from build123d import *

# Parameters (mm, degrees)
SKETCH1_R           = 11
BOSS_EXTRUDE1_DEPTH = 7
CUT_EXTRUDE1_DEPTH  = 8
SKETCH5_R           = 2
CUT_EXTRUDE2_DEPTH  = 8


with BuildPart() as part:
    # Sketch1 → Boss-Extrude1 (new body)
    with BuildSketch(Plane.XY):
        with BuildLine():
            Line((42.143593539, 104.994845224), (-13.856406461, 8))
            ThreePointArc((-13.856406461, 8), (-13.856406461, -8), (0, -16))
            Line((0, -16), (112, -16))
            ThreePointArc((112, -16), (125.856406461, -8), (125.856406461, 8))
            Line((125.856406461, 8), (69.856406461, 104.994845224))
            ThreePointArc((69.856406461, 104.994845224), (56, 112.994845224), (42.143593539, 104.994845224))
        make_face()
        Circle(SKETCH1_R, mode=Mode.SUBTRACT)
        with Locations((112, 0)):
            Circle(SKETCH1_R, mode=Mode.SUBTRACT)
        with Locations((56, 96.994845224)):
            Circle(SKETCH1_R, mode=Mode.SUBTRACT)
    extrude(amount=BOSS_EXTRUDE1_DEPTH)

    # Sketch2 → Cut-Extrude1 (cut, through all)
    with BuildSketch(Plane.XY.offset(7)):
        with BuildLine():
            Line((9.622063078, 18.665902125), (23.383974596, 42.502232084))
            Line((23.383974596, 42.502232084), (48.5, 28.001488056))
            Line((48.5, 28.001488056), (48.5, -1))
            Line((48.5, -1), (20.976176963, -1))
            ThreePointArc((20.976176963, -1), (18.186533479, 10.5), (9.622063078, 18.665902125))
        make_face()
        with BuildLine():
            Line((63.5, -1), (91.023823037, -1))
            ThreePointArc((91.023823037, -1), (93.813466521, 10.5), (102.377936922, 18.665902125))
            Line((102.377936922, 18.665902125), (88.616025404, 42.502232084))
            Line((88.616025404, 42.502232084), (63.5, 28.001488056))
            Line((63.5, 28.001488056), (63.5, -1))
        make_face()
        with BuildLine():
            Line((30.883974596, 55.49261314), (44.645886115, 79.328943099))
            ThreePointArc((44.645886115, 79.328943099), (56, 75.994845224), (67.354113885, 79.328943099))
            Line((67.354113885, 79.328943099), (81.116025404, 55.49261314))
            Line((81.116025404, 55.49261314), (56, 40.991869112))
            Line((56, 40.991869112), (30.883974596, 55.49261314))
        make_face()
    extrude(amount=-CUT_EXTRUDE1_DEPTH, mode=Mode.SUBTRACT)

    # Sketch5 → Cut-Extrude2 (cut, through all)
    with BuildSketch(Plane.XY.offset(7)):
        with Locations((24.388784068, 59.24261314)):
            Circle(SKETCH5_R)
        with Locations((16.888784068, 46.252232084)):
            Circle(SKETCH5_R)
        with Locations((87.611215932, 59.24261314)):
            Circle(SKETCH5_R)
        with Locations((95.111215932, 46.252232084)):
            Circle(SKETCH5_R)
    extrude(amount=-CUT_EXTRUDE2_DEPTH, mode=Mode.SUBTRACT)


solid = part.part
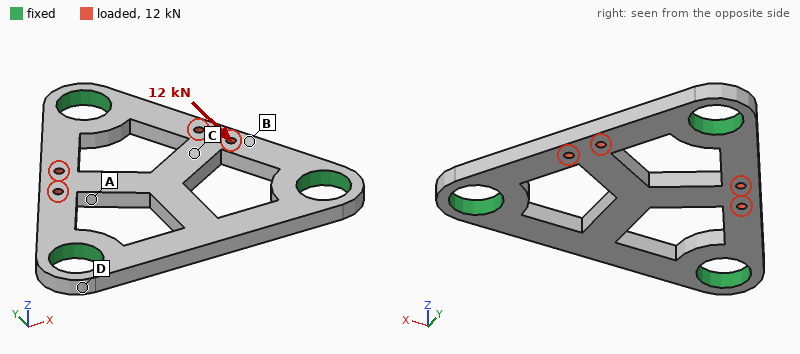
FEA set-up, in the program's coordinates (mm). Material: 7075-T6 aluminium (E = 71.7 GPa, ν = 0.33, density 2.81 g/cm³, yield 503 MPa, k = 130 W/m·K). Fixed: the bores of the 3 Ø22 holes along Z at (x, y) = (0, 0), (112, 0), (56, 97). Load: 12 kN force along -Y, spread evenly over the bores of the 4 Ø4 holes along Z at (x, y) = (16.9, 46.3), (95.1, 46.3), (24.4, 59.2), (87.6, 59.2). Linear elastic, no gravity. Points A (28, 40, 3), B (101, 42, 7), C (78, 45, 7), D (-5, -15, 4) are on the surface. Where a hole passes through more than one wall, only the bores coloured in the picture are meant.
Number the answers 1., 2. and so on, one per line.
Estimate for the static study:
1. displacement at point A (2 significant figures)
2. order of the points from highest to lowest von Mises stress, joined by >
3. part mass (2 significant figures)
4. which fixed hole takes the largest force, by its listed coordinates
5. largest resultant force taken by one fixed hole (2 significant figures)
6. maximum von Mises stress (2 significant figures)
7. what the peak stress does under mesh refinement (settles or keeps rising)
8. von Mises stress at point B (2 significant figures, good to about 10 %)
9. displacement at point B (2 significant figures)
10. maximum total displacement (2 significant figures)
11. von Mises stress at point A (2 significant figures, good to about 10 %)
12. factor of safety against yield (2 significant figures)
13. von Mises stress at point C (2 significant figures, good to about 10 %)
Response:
1. 29 µm
2. B > A > C > D
3. 140 g
4. (56, 97)
5. 4.9 kN
6. 78 MPa
7. settles
8. 34 MPa
9. 21 µm
10. 38 µm
11. 26 MPa
12. 6.4
13. 19 MPa
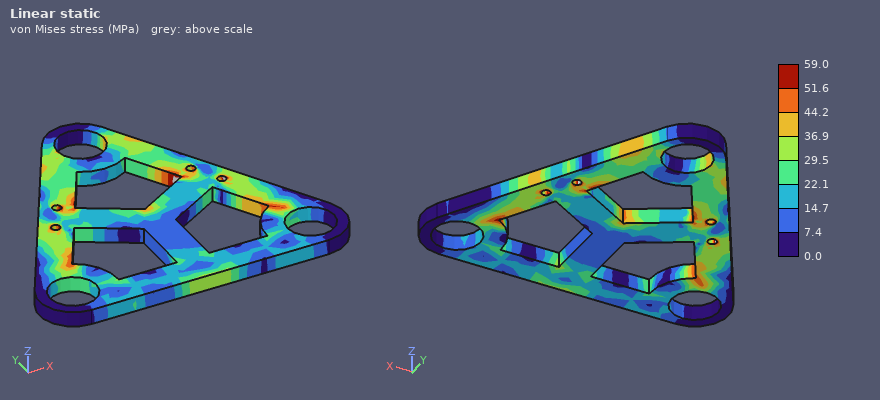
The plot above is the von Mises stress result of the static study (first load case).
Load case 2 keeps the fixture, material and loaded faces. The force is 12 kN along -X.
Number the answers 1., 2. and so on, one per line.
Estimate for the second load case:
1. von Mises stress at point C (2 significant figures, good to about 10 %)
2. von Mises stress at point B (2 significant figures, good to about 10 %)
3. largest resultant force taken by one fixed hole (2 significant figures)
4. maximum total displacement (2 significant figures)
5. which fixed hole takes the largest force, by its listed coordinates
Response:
1. 27 MPa
2. 48 MPa
3. 5.4 kN
4. 99 µm
5. (56, 97)
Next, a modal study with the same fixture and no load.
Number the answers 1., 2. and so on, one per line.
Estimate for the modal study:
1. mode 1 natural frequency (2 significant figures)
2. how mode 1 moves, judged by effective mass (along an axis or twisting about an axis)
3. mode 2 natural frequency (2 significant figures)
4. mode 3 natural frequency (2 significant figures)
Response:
1. 2900 Hz
2. along Z
3. 4200 Hz
4. 4200 Hz
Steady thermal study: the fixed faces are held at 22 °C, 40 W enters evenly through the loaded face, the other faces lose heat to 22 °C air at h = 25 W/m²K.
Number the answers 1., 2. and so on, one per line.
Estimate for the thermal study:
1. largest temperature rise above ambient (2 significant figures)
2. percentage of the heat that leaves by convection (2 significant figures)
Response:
1. 24 K
2. 11 %
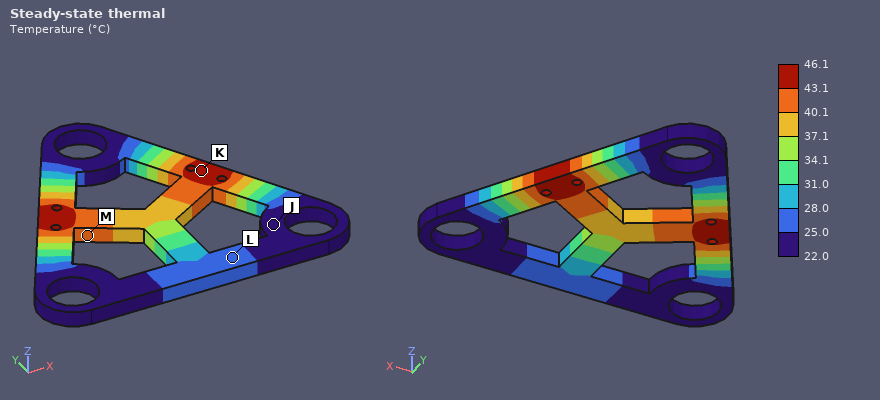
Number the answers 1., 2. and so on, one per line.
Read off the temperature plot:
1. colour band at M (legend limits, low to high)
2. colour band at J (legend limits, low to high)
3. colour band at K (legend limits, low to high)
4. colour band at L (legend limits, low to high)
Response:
1. 40.1 to 43.1 °C
2. 22.0 to 25.0 °C
3. 43.1 to 46.1 °C
4. 25.0 to 28.0 °C
